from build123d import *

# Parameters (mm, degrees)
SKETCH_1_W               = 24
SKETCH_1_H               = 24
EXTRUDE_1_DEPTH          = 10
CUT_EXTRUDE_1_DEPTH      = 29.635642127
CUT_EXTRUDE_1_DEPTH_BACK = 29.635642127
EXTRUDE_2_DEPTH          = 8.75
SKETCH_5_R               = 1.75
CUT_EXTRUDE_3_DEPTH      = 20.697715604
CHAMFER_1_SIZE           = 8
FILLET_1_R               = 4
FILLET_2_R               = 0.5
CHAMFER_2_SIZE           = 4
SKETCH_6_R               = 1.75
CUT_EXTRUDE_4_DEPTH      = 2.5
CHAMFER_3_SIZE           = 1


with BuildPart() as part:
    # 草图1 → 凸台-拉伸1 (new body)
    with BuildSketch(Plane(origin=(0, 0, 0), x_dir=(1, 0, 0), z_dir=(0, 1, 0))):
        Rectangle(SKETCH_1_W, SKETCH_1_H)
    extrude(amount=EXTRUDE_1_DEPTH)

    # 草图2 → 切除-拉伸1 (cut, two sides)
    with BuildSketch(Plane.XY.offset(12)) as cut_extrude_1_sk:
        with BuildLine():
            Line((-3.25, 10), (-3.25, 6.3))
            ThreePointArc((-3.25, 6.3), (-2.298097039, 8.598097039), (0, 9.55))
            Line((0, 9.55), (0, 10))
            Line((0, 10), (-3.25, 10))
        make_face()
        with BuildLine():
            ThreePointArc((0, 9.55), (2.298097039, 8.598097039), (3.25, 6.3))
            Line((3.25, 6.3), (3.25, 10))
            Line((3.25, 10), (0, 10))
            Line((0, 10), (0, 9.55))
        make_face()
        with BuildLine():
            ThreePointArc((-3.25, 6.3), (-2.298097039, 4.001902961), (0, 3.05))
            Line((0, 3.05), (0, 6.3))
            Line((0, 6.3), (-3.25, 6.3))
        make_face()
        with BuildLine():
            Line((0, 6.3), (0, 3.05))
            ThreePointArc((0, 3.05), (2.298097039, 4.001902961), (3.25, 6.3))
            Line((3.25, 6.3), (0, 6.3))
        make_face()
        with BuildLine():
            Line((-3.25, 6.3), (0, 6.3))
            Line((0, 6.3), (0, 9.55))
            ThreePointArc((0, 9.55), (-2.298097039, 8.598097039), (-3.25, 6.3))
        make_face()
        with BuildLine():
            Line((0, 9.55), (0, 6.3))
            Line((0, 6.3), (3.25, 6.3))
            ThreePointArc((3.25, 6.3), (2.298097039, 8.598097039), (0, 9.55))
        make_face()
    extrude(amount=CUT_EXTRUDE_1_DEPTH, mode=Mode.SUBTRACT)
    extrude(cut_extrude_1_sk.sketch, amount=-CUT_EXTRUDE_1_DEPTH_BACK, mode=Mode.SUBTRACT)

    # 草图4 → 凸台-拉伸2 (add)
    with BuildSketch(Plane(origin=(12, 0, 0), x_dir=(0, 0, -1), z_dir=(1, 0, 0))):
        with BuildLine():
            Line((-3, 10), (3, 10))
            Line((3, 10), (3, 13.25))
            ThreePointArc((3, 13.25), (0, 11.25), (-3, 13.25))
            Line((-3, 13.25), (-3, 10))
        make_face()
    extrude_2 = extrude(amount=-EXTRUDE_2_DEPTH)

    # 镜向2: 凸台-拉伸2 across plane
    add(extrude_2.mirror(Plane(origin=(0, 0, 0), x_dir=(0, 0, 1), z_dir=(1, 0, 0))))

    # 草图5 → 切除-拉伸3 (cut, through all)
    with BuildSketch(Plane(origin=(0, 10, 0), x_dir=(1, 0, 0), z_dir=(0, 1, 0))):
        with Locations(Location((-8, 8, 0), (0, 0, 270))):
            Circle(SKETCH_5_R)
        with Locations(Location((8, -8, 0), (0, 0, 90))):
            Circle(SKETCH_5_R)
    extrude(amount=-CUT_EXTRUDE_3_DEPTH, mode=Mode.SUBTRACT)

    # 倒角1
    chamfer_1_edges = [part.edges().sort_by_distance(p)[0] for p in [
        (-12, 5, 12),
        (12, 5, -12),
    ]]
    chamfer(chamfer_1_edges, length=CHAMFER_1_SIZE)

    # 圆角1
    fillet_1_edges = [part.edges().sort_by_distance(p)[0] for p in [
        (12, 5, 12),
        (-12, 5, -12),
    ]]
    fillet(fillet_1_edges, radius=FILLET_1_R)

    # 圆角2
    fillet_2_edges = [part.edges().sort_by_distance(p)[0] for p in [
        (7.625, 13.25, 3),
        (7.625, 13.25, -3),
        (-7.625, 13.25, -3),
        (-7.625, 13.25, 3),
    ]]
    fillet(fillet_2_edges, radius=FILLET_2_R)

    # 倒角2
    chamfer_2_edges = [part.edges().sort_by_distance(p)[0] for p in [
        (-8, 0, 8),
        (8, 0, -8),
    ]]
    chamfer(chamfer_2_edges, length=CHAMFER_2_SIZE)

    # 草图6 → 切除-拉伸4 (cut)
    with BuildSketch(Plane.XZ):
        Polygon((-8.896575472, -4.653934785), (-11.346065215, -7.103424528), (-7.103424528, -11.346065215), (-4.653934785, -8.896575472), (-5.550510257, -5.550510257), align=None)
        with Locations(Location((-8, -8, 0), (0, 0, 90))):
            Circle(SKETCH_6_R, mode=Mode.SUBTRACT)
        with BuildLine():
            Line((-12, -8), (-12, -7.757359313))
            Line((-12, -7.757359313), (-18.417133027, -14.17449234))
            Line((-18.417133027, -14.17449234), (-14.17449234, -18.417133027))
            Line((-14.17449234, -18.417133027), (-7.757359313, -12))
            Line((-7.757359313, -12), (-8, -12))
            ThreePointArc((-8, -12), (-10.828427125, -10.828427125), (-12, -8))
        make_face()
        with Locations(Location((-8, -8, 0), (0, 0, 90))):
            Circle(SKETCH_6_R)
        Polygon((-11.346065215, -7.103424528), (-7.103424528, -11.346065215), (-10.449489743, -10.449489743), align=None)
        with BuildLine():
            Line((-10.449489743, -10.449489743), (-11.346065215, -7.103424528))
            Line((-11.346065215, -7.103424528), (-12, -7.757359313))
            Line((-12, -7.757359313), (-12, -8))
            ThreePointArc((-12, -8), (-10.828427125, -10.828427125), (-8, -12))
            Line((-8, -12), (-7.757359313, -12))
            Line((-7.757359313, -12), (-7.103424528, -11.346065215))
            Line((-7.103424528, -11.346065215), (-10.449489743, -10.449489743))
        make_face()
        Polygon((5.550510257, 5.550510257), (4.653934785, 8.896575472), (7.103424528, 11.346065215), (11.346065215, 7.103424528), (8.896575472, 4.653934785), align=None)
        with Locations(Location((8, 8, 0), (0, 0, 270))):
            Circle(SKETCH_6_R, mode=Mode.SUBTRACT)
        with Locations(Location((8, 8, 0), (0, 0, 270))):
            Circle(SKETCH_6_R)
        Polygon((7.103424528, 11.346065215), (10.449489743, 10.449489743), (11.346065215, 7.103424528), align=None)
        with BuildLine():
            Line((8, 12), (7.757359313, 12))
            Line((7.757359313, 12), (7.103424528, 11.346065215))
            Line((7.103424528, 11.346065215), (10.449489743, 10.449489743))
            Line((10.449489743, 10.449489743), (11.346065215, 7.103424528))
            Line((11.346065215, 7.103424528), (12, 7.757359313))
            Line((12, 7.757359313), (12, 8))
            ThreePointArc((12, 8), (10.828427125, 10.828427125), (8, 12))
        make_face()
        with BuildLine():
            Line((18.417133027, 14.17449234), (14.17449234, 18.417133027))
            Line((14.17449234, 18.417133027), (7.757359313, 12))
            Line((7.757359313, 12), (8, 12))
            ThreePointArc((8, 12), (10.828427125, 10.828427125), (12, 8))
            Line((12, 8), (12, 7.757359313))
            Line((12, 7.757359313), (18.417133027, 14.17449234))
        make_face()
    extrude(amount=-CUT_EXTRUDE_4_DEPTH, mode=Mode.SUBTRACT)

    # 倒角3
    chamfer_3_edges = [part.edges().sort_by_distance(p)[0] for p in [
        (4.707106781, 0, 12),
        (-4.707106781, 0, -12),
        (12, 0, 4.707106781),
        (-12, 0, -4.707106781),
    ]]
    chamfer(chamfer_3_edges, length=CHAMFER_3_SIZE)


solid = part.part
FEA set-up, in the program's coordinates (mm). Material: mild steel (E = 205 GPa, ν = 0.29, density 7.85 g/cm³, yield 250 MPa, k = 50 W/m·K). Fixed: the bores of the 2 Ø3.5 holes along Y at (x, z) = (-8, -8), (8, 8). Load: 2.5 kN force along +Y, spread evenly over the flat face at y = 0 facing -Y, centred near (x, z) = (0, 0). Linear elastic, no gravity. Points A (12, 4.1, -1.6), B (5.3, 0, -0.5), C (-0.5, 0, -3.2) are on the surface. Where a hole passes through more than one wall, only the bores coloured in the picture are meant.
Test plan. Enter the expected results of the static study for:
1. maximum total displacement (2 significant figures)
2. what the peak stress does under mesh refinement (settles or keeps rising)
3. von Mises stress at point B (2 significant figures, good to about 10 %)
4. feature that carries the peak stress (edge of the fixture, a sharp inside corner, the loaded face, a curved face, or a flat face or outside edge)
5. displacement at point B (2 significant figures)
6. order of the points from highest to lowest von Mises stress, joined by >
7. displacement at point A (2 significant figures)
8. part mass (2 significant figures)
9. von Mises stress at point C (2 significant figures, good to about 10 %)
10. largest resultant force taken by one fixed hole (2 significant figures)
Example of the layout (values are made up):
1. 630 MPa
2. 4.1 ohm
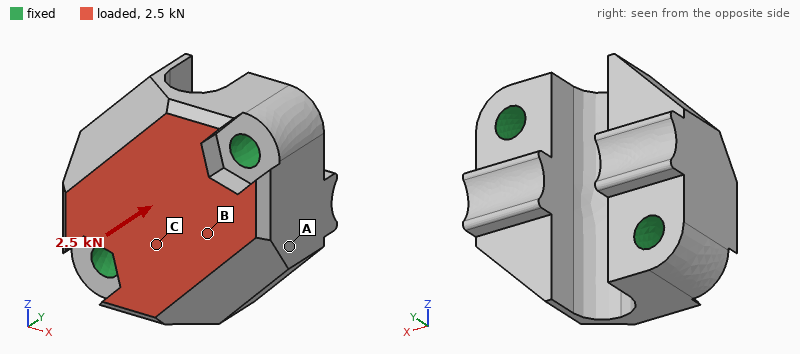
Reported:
1. 3.3 µm
2. keeps rising
3. 15 MPa
4. edge of the fixture
5. 2.1 µm
6. C > B > A
7. 1.5 µm
8. 29 g
9. 31 MPa
10. 1.4 kN
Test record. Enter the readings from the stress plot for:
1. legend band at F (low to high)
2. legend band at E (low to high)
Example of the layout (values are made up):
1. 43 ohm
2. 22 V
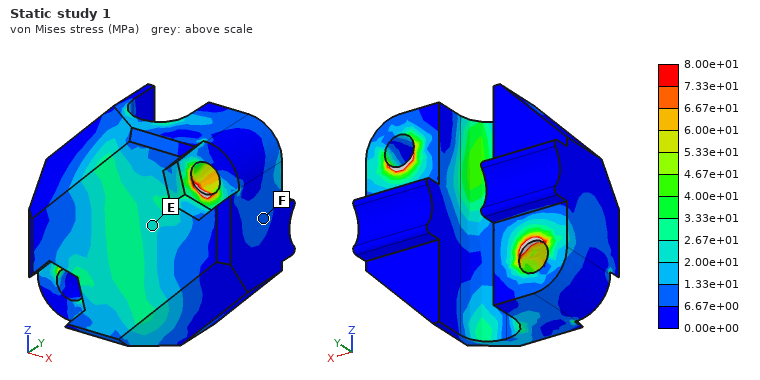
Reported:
1. 6.67e+00 to 1.33e+01 MPa
2. 2.00e+01 to 2.67e+01 MPa
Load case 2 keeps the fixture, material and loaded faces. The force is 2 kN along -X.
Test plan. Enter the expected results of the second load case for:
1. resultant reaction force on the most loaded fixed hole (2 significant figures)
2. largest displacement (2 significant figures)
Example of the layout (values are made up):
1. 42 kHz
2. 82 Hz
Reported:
1. 1.1 kN
2. 3.2 µm
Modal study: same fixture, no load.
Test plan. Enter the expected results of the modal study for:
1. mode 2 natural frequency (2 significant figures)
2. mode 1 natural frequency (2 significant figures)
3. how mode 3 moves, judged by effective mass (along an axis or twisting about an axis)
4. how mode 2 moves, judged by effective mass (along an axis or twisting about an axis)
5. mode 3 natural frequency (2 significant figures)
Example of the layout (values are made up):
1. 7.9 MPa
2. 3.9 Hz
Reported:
1. 29 kHz
2. 25 kHz
3. along X
4. along Y
5. 34 kHz
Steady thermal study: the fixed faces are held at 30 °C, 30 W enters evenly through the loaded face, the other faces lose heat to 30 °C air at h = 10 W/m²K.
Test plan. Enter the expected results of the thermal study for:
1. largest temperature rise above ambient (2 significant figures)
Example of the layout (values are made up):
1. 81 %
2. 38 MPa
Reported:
1. 29 K
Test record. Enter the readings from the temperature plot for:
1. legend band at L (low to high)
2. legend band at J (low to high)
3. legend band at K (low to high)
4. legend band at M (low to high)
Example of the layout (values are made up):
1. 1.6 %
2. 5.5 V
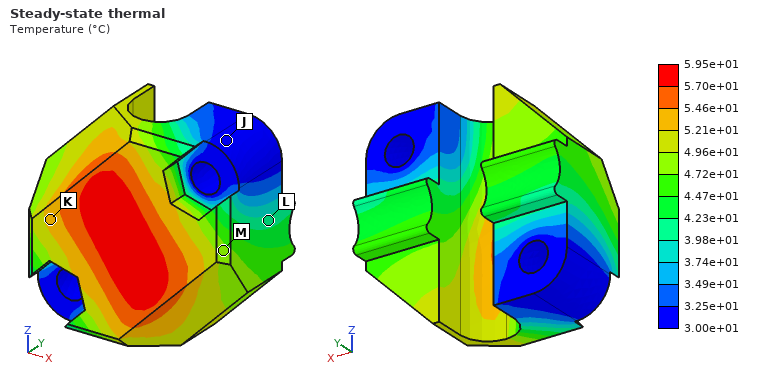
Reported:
1. 3.98e+01 to 4.23e+01 °C
2. 3.00e+01 to 3.25e+01 °C
3. 5.21e+01 to 5.46e+01 °C
4. 4.72e+01 to 4.96e+01 °C
